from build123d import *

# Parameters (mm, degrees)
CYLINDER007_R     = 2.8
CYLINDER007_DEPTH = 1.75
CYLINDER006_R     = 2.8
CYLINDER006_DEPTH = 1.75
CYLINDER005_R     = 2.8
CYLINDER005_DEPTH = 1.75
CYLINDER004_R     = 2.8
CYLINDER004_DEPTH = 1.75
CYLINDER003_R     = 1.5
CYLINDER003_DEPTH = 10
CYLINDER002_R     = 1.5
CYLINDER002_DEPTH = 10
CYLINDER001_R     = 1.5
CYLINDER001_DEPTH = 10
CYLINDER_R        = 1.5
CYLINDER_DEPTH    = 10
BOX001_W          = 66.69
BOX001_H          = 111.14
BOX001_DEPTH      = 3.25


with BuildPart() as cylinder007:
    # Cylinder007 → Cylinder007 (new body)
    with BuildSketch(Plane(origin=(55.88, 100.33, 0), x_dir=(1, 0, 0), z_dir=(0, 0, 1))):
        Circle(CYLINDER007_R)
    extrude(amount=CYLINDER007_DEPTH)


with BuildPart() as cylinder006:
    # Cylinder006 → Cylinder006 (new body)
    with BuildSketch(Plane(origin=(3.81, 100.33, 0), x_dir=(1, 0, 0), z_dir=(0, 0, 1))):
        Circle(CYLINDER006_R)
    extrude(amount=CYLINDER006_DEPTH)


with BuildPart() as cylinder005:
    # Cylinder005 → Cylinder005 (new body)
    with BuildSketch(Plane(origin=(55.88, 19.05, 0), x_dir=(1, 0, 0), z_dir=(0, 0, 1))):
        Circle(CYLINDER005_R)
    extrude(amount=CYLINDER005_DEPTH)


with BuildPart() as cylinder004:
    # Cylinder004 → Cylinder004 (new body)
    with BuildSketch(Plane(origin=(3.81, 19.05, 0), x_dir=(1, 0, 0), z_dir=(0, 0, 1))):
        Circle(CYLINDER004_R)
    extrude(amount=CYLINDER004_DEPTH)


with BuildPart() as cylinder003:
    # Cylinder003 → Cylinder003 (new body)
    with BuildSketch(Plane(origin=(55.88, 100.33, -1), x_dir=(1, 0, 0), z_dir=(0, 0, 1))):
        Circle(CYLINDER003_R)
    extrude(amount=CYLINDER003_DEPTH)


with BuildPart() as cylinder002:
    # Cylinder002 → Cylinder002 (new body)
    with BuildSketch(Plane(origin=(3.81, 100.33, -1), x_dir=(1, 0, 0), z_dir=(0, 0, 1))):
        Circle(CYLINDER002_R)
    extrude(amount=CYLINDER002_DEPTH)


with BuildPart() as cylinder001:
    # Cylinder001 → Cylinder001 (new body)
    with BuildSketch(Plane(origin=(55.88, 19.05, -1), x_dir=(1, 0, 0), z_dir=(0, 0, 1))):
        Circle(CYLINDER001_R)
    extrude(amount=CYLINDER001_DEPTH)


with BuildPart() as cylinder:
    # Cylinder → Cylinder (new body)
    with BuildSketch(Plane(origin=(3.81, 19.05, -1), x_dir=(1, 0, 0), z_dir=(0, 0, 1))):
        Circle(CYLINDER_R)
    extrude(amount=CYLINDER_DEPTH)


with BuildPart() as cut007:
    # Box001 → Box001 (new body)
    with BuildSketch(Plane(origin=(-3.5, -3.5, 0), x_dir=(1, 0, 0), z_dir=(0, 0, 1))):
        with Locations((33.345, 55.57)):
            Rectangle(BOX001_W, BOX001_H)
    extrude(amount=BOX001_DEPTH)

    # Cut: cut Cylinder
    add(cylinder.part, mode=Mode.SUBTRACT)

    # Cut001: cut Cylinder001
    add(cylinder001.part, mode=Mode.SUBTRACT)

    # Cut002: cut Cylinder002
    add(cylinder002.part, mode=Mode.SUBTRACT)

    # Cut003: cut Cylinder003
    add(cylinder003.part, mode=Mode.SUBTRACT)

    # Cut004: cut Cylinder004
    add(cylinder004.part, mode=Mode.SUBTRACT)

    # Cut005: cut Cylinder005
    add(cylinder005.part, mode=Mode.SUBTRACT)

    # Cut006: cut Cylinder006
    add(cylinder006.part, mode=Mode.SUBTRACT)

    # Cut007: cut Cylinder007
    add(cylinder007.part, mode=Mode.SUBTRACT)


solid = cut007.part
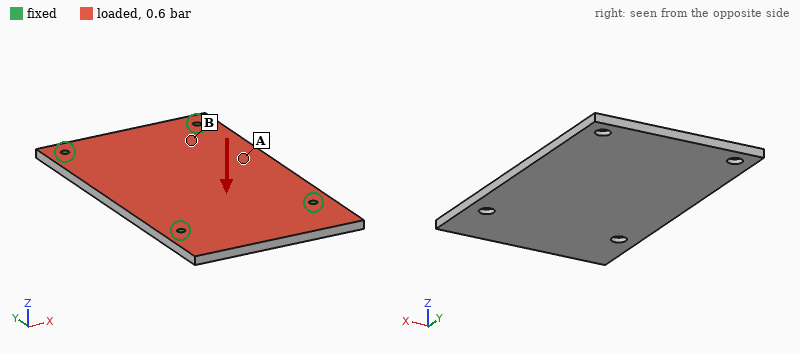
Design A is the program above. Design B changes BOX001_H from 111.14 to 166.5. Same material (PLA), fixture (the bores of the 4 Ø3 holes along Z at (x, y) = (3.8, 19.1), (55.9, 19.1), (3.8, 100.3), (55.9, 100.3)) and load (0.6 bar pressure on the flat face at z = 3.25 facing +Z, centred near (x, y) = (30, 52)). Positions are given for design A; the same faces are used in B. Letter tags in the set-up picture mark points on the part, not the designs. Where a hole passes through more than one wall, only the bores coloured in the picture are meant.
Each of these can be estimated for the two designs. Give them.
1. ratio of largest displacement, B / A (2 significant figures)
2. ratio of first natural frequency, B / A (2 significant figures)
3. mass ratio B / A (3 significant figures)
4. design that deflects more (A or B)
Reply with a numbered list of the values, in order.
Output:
1. 5.8
2. 0.45
3. 1.50
4. B
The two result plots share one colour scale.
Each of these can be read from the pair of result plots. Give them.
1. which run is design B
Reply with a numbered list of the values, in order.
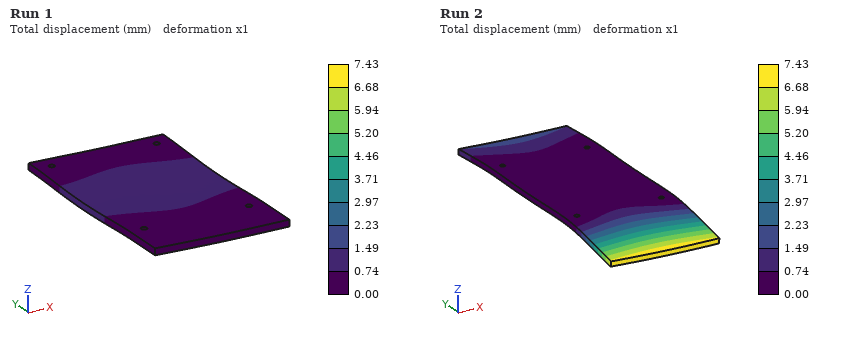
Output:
1. Run 2
